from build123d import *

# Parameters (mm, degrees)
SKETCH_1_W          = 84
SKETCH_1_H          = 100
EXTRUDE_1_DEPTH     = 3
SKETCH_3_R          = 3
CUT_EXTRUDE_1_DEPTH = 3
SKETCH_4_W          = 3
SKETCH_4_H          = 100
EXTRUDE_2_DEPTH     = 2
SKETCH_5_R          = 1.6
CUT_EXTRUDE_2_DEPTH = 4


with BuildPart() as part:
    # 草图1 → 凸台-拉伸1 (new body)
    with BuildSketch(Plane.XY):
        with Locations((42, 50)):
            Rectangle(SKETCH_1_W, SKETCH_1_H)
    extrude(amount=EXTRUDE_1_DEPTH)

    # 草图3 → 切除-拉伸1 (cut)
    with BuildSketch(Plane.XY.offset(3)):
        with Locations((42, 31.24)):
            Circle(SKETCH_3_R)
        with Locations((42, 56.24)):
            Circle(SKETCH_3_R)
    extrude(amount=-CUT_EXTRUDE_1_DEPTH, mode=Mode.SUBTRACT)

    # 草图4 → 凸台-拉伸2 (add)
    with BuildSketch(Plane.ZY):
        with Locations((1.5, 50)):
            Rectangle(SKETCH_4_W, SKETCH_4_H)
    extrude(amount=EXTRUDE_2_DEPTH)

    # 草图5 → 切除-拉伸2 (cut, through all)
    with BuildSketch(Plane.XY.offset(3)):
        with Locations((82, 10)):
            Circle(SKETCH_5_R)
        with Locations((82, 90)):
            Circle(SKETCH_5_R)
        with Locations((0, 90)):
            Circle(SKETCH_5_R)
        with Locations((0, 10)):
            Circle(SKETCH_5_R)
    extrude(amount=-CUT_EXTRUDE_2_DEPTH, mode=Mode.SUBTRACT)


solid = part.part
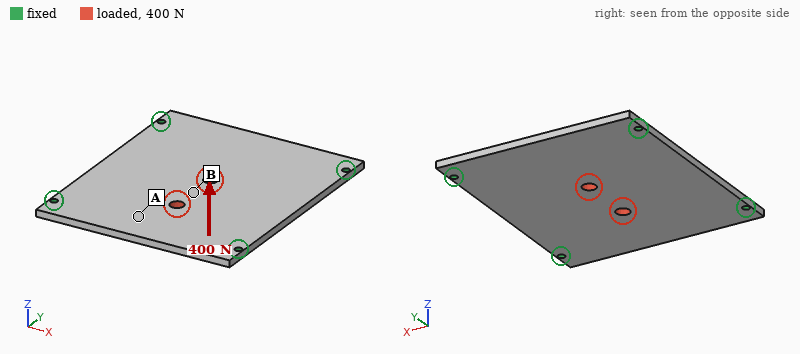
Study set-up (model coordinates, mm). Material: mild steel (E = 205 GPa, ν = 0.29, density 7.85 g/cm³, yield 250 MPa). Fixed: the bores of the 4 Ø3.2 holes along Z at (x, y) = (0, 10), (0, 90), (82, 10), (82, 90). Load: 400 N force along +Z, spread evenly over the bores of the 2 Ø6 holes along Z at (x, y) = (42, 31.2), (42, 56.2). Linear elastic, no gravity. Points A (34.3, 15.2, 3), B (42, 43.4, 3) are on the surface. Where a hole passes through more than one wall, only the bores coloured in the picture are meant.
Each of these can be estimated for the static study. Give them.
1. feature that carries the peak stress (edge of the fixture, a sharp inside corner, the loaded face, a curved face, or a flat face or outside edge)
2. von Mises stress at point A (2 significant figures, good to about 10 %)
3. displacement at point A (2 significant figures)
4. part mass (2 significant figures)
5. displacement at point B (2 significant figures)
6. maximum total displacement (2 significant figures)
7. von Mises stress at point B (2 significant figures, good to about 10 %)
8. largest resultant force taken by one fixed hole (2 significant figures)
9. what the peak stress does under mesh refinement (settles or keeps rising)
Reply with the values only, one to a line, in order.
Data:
edge of the fixture
27 MPa
45 µm
200 g
80 µm
81 µm
44 MPa
120 N
keeps rising
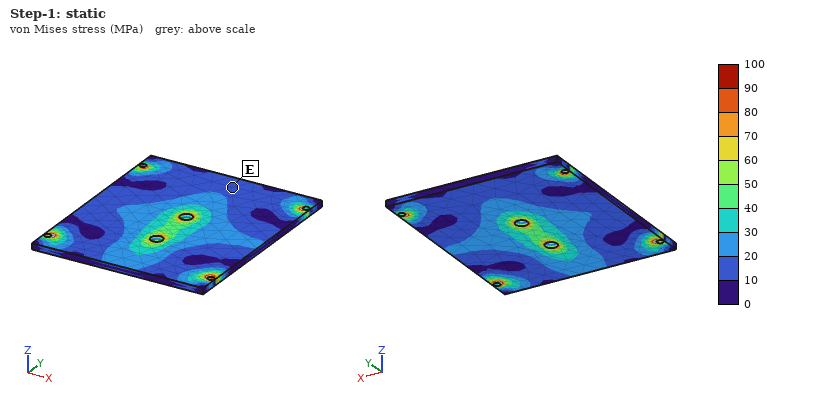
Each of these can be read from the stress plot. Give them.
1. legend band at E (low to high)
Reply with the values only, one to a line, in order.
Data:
10 to 20 MPa
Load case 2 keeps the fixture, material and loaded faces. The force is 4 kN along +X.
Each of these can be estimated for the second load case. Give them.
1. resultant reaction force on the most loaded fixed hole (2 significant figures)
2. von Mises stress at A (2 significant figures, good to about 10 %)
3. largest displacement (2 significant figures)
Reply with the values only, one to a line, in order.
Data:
1.2 kN
11 MPa
6.3 µm
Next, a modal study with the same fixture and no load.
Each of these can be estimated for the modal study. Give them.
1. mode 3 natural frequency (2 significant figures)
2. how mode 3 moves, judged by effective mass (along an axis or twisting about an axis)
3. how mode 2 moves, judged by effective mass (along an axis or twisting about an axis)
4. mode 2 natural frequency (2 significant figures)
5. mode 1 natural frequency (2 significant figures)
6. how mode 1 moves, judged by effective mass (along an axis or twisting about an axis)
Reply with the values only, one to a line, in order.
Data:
2600 Hz
twisting about Y
twisting about X
2400 Hz
1400 Hz
along Z
